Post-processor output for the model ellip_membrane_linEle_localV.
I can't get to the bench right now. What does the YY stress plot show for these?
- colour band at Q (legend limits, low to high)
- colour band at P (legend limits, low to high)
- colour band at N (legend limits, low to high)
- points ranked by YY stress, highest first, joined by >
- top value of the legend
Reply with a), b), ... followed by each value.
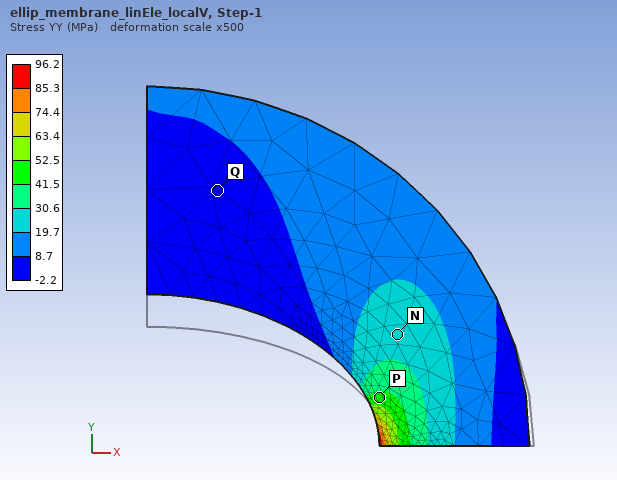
a) -2.2 to 8.7 MPa
b) 41.5 to 52.5 MPa
c) 19.7 to 30.6 MPa
d) P > N > Q
e) 96.2 MPa
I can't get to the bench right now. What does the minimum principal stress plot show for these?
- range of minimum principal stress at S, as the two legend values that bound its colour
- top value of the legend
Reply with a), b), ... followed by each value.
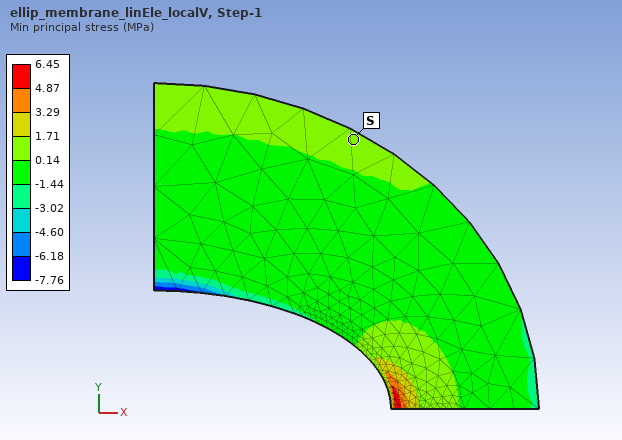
a) 0.14 to 1.71 MPa
b) 6.45 MPa
